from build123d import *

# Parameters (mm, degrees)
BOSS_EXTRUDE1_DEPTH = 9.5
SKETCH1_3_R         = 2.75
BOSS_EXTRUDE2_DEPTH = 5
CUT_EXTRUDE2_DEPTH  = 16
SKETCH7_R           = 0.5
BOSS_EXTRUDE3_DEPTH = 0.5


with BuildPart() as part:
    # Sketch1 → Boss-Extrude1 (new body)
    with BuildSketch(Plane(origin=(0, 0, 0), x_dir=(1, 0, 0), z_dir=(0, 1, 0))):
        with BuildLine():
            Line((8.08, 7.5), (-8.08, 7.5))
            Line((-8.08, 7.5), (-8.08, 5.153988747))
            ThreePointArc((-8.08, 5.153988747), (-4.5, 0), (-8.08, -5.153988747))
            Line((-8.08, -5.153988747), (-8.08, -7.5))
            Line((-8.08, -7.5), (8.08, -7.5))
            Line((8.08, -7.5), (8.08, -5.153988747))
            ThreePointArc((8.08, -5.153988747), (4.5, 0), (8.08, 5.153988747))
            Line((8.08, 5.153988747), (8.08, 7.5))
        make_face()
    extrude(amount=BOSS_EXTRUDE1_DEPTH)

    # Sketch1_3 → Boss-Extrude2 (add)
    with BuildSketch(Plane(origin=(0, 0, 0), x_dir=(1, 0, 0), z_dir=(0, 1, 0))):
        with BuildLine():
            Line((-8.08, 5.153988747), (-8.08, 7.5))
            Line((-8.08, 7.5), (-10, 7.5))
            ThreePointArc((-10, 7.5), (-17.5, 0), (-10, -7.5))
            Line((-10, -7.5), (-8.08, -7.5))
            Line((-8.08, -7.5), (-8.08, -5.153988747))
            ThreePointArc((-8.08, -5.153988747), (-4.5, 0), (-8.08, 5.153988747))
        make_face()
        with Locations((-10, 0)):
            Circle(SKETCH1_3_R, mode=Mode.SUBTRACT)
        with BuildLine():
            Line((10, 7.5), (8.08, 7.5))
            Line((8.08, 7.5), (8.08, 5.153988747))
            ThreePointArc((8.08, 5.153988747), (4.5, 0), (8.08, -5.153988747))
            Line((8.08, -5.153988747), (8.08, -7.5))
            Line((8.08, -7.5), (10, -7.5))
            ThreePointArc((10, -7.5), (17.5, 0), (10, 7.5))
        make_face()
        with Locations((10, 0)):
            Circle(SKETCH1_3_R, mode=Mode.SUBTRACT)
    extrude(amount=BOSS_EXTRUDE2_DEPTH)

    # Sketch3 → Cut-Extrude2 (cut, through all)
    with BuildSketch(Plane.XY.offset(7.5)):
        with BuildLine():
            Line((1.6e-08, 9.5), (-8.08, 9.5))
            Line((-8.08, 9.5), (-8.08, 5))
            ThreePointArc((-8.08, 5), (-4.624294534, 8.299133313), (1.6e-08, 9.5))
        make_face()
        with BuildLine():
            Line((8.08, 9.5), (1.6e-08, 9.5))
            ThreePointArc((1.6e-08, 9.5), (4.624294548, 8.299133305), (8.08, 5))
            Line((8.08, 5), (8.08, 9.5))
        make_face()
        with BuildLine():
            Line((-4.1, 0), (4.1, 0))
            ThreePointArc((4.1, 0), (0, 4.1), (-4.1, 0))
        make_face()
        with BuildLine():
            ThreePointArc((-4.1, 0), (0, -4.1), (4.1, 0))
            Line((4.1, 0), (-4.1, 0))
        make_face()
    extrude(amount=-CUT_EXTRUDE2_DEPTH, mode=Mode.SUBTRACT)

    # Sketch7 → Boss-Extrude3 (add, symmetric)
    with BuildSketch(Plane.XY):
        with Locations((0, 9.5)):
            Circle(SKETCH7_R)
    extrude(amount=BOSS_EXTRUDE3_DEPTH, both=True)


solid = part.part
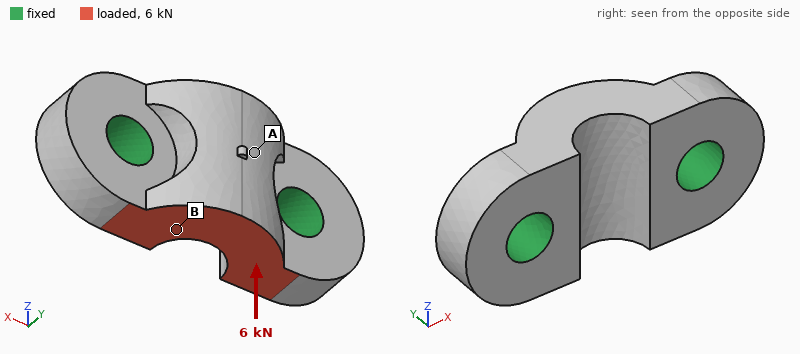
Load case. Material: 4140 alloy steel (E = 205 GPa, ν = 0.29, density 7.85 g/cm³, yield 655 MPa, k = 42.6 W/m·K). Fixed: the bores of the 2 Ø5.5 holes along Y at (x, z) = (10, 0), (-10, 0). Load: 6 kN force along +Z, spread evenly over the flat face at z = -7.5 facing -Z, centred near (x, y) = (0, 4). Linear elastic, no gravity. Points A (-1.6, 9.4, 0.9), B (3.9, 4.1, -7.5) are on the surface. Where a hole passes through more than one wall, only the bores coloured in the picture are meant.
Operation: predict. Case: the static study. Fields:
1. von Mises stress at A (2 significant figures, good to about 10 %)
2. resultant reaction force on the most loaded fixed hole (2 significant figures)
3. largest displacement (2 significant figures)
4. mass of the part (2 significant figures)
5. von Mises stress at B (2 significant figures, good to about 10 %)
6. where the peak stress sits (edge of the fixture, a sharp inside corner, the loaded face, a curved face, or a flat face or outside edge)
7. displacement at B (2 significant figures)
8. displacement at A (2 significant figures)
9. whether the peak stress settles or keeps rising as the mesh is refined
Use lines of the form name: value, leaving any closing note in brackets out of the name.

von Mises stress at A: 27 MPa
resultant reaction force on the most loaded fixed hole: 3.0 kN
largest displacement: 11 µm
mass of the part: 19 g
von Mises stress at B: 73 MPa
where the peak stress sits: edge of the fixture
displacement at B: 6.6 µm
displacement at A: 7.1 µm
whether the peak stress settles or keeps rising as the mesh is refined: keeps rising
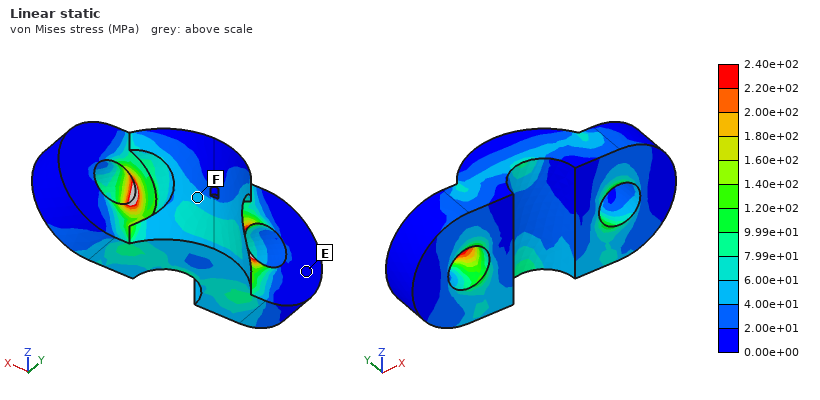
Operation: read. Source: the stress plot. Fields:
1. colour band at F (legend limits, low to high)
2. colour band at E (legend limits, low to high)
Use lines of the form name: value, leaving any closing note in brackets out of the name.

colour band at F: 4.00e+01 to 6.00e+01 MPa
colour band at E: 0.00e+00 to 2.00e+01 MPa
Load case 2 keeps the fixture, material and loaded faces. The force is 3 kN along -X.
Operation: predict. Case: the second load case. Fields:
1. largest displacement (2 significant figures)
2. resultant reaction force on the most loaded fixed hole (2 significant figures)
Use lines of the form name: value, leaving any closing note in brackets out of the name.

largest displacement: 3.7 µm
resultant reaction force on the most loaded fixed hole: 1.7 kN
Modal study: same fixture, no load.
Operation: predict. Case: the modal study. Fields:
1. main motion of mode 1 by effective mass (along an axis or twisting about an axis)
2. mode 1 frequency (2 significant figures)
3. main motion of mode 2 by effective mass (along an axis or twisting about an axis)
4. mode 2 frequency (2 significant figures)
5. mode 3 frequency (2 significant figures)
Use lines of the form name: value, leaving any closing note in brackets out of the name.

main motion of mode 1 by effective mass: along Z
mode 1 frequency: 39 kHz
main motion of mode 2 by effective mass: along Y
mode 2 frequency: 58 kHz
mode 3 frequency: 77 kHz
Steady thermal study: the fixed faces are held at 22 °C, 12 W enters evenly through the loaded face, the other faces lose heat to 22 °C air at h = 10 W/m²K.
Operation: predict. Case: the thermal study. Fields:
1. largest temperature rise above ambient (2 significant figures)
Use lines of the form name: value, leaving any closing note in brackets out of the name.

largest temperature rise above ambient: 21 K
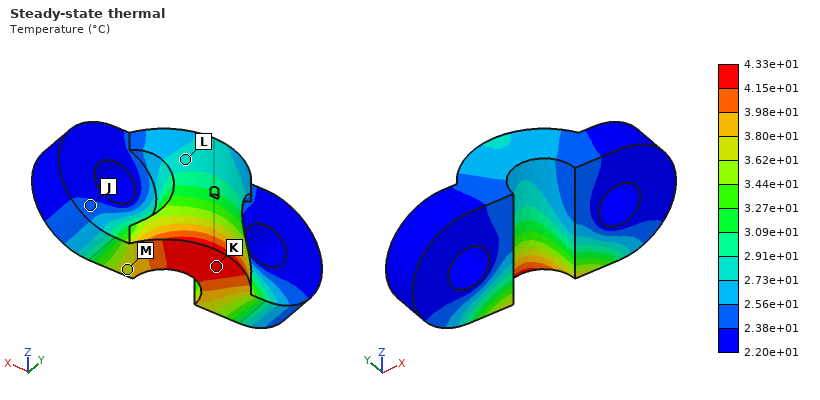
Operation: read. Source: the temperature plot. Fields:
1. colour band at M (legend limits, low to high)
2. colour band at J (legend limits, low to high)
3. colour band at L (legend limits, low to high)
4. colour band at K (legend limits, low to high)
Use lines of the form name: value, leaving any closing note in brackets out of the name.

colour band at M: 3.62e+01 to 3.80e+01 °C
colour band at J: 2.38e+01 to 2.56e+01 °C
colour band at L: 2.73e+01 to 2.91e+01 °C
colour band at K: 4.15e+01 to 4.33e+01 °C
